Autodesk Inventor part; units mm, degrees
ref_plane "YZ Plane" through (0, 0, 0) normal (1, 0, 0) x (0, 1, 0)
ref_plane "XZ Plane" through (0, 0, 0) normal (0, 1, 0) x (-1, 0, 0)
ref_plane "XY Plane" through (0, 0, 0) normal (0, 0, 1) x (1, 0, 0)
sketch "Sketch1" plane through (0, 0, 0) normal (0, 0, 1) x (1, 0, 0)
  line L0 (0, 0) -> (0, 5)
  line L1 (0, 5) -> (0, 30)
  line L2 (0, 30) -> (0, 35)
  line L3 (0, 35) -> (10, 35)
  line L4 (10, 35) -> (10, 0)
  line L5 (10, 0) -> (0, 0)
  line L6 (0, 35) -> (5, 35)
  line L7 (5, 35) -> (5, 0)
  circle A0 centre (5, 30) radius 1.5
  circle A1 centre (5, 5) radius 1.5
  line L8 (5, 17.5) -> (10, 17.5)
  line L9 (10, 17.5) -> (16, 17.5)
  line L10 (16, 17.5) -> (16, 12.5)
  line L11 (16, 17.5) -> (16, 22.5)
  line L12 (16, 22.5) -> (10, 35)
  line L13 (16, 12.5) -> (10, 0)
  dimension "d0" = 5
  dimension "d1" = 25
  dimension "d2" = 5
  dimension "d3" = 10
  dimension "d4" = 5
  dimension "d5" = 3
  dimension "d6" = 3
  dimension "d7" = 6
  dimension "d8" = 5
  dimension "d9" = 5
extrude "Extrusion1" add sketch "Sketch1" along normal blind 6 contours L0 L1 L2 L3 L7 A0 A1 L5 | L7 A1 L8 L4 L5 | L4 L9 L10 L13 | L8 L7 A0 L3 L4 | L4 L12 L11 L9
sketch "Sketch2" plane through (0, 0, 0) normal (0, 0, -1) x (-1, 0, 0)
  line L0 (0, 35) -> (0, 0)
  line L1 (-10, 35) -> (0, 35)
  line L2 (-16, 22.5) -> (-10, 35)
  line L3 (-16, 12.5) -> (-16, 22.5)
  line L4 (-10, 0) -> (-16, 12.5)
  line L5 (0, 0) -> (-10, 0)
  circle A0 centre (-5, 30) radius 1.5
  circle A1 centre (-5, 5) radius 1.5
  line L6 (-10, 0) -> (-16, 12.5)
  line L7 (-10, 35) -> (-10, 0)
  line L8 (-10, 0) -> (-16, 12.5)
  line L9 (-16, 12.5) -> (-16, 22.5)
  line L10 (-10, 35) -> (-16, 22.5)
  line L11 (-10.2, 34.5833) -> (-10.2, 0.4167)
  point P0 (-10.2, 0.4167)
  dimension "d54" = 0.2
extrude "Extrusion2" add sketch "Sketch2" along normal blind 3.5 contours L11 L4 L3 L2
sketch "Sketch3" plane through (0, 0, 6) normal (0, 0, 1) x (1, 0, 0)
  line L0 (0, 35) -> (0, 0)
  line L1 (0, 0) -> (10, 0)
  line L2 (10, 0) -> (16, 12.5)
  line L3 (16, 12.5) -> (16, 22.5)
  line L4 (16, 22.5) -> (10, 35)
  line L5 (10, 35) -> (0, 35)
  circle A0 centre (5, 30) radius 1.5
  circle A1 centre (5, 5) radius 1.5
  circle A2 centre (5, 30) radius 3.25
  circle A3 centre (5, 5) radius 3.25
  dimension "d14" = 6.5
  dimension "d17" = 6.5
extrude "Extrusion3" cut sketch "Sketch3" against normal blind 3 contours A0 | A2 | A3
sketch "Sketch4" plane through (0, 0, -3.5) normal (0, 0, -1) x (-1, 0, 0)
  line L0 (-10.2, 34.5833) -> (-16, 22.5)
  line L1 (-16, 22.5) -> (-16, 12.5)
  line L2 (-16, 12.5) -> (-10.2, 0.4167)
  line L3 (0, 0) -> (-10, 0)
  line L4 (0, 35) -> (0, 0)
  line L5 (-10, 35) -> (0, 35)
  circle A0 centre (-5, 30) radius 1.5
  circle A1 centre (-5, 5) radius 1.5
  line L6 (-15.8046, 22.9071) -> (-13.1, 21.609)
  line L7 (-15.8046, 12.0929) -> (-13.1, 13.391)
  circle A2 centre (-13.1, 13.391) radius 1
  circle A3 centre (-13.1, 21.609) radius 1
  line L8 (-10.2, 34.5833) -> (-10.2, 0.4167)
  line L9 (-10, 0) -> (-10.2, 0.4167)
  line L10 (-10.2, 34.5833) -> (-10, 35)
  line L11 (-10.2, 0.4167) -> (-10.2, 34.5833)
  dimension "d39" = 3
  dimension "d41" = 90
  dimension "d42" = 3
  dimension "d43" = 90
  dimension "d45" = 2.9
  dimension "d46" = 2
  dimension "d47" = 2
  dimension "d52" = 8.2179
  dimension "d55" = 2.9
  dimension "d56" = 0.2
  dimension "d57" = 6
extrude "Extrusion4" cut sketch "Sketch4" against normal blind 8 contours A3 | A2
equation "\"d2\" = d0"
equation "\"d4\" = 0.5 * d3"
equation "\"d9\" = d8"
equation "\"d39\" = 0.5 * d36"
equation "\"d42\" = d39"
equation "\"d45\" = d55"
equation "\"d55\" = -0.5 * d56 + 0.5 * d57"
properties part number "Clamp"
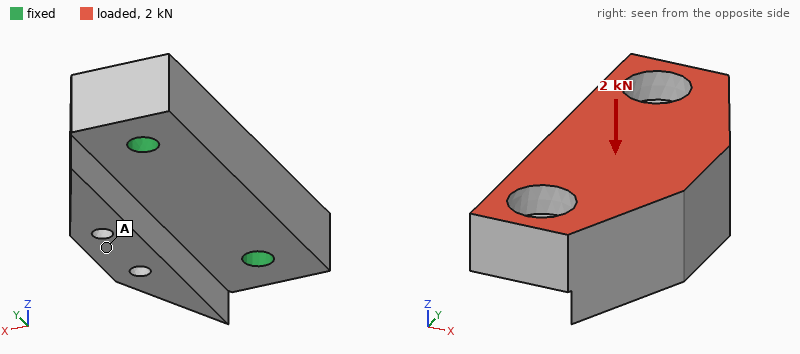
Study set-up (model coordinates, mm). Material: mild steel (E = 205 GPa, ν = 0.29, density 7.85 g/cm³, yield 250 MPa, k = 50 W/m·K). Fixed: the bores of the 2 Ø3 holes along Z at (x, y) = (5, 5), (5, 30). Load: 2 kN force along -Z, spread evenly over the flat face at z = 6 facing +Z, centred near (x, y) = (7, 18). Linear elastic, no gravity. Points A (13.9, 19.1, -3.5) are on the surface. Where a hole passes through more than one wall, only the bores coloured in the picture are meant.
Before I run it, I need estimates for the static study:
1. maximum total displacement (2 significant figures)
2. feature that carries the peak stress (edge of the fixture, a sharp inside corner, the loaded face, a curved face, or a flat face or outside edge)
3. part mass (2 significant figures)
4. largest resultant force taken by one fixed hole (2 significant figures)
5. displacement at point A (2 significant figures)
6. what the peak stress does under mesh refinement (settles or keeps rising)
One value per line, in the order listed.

11 µm
edge of the fixture
24 g
1.0 kN
9.7 µm
keeps rising
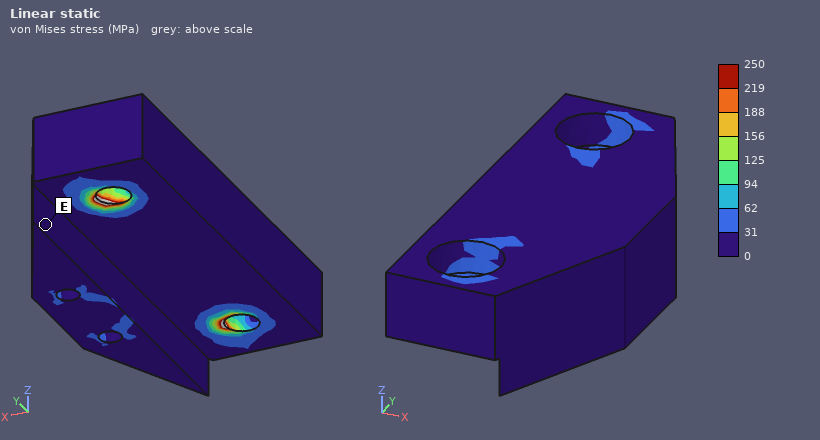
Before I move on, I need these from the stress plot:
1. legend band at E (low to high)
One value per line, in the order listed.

0 to 31 MPa
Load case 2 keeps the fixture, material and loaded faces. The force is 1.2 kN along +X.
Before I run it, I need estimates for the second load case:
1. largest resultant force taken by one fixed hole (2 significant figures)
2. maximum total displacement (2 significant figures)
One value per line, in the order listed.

620 N
9.2 µm
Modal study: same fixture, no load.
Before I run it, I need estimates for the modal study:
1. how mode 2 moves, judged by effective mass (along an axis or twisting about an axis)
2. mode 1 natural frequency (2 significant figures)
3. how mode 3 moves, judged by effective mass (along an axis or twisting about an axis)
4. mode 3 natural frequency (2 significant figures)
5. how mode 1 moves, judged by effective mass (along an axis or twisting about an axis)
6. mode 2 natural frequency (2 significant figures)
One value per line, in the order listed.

along Z
15 kHz
along X
36 kHz
along Z
31 kHz
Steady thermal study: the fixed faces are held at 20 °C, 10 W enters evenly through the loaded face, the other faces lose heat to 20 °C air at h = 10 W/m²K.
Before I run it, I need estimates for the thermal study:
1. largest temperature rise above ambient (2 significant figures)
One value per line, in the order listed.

13 K
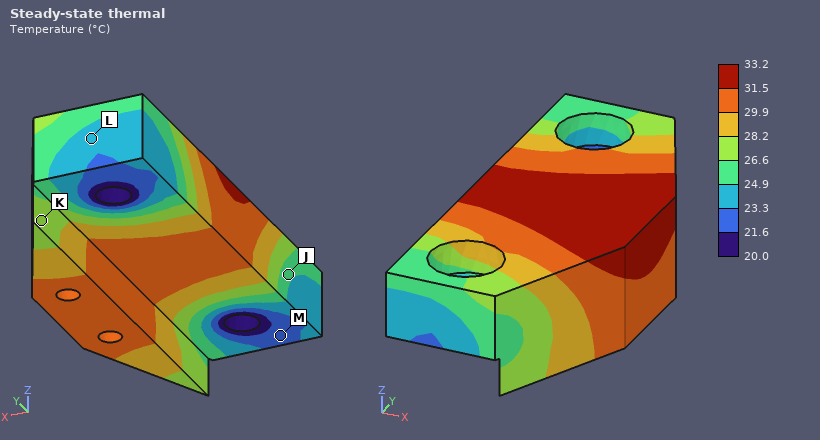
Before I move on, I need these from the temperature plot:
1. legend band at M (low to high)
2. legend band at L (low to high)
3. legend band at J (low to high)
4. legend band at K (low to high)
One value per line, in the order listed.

21.6 to 23.3 °C
23.3 to 24.9 °C
24.9 to 26.6 °C
26.6 to 28.2 °C
